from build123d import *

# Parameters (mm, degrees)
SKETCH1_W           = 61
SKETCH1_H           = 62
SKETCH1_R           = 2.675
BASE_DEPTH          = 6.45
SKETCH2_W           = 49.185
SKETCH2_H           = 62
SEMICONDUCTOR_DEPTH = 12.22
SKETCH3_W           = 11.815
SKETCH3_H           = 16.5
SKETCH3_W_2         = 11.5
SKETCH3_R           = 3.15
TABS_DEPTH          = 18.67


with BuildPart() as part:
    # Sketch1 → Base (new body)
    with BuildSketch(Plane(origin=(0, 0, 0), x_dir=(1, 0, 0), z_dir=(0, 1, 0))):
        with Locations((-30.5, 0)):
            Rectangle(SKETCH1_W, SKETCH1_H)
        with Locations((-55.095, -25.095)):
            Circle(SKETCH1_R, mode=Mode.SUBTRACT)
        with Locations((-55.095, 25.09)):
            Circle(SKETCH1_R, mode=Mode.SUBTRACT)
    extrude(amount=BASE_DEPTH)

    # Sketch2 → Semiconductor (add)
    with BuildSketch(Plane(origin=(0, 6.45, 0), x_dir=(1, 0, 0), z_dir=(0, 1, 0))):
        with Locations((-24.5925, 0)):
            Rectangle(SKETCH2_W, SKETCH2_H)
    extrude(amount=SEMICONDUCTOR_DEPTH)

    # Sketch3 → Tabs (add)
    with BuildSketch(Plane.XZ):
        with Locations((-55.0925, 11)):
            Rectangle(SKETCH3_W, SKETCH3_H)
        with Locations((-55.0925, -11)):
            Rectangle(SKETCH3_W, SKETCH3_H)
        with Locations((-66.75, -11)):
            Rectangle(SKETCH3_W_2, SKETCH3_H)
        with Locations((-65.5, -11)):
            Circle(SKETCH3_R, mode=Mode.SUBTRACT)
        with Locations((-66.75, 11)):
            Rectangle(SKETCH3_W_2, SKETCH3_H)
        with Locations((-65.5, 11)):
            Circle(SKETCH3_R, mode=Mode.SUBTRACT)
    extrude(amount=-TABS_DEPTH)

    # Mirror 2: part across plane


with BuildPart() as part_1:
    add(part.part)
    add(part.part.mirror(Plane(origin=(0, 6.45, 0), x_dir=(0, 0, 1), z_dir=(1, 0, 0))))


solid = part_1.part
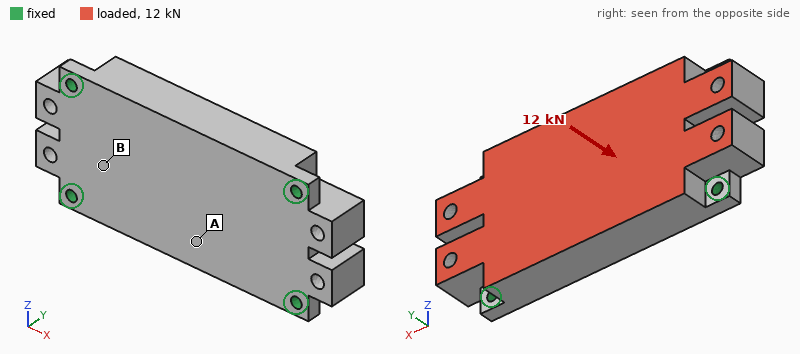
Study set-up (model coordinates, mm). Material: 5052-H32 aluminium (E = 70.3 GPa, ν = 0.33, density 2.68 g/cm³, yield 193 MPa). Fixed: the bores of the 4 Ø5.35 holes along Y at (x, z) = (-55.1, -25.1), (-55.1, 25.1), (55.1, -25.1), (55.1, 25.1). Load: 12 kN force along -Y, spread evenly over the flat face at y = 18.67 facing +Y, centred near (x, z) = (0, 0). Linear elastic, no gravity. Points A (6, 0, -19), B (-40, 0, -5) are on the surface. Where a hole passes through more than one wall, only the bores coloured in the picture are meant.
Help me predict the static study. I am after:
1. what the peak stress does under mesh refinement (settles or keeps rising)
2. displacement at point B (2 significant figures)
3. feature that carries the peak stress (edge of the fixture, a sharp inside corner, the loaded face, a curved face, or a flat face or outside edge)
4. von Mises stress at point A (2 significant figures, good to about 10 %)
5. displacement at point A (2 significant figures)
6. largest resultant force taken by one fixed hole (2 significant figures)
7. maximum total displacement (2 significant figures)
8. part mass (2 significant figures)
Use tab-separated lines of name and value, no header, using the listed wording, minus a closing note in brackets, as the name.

what the peak stress does under mesh refinement	keeps rising
displacement at point B	26 µm
feature that carries the peak stress	edge of the fixture
von Mises stress at point A	18 MPa
displacement at point A	49 µm
largest resultant force taken by one fixed hole	4.0 kN
maximum total displacement	52 µm
part mass	390 g
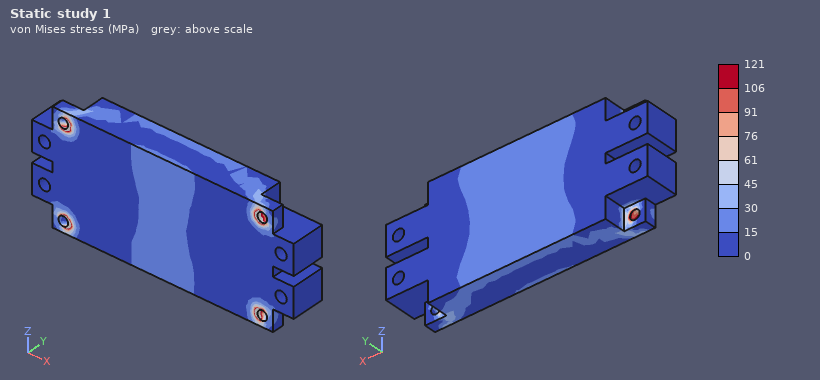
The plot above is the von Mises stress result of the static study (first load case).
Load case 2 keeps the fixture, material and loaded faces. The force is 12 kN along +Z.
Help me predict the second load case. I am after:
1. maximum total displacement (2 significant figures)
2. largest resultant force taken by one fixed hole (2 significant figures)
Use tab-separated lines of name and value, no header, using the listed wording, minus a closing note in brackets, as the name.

maximum total displacement	26 µm
largest resultant force taken by one fixed hole	4.0 kN
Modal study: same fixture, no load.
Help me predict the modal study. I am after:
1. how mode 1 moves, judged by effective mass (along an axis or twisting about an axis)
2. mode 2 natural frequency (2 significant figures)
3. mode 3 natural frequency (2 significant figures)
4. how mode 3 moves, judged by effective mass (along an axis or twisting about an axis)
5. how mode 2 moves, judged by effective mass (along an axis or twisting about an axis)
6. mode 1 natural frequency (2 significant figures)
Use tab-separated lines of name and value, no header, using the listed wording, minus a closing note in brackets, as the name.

how mode 1 moves, judged by effective mass	along Y
mode 2 natural frequency	7400 Hz
mode 3 natural frequency	8800 Hz
how mode 3 moves, judged by effective mass	along Z
how mode 2 moves, judged by effective mass	twisting about X
mode 1 natural frequency	4400 Hz
